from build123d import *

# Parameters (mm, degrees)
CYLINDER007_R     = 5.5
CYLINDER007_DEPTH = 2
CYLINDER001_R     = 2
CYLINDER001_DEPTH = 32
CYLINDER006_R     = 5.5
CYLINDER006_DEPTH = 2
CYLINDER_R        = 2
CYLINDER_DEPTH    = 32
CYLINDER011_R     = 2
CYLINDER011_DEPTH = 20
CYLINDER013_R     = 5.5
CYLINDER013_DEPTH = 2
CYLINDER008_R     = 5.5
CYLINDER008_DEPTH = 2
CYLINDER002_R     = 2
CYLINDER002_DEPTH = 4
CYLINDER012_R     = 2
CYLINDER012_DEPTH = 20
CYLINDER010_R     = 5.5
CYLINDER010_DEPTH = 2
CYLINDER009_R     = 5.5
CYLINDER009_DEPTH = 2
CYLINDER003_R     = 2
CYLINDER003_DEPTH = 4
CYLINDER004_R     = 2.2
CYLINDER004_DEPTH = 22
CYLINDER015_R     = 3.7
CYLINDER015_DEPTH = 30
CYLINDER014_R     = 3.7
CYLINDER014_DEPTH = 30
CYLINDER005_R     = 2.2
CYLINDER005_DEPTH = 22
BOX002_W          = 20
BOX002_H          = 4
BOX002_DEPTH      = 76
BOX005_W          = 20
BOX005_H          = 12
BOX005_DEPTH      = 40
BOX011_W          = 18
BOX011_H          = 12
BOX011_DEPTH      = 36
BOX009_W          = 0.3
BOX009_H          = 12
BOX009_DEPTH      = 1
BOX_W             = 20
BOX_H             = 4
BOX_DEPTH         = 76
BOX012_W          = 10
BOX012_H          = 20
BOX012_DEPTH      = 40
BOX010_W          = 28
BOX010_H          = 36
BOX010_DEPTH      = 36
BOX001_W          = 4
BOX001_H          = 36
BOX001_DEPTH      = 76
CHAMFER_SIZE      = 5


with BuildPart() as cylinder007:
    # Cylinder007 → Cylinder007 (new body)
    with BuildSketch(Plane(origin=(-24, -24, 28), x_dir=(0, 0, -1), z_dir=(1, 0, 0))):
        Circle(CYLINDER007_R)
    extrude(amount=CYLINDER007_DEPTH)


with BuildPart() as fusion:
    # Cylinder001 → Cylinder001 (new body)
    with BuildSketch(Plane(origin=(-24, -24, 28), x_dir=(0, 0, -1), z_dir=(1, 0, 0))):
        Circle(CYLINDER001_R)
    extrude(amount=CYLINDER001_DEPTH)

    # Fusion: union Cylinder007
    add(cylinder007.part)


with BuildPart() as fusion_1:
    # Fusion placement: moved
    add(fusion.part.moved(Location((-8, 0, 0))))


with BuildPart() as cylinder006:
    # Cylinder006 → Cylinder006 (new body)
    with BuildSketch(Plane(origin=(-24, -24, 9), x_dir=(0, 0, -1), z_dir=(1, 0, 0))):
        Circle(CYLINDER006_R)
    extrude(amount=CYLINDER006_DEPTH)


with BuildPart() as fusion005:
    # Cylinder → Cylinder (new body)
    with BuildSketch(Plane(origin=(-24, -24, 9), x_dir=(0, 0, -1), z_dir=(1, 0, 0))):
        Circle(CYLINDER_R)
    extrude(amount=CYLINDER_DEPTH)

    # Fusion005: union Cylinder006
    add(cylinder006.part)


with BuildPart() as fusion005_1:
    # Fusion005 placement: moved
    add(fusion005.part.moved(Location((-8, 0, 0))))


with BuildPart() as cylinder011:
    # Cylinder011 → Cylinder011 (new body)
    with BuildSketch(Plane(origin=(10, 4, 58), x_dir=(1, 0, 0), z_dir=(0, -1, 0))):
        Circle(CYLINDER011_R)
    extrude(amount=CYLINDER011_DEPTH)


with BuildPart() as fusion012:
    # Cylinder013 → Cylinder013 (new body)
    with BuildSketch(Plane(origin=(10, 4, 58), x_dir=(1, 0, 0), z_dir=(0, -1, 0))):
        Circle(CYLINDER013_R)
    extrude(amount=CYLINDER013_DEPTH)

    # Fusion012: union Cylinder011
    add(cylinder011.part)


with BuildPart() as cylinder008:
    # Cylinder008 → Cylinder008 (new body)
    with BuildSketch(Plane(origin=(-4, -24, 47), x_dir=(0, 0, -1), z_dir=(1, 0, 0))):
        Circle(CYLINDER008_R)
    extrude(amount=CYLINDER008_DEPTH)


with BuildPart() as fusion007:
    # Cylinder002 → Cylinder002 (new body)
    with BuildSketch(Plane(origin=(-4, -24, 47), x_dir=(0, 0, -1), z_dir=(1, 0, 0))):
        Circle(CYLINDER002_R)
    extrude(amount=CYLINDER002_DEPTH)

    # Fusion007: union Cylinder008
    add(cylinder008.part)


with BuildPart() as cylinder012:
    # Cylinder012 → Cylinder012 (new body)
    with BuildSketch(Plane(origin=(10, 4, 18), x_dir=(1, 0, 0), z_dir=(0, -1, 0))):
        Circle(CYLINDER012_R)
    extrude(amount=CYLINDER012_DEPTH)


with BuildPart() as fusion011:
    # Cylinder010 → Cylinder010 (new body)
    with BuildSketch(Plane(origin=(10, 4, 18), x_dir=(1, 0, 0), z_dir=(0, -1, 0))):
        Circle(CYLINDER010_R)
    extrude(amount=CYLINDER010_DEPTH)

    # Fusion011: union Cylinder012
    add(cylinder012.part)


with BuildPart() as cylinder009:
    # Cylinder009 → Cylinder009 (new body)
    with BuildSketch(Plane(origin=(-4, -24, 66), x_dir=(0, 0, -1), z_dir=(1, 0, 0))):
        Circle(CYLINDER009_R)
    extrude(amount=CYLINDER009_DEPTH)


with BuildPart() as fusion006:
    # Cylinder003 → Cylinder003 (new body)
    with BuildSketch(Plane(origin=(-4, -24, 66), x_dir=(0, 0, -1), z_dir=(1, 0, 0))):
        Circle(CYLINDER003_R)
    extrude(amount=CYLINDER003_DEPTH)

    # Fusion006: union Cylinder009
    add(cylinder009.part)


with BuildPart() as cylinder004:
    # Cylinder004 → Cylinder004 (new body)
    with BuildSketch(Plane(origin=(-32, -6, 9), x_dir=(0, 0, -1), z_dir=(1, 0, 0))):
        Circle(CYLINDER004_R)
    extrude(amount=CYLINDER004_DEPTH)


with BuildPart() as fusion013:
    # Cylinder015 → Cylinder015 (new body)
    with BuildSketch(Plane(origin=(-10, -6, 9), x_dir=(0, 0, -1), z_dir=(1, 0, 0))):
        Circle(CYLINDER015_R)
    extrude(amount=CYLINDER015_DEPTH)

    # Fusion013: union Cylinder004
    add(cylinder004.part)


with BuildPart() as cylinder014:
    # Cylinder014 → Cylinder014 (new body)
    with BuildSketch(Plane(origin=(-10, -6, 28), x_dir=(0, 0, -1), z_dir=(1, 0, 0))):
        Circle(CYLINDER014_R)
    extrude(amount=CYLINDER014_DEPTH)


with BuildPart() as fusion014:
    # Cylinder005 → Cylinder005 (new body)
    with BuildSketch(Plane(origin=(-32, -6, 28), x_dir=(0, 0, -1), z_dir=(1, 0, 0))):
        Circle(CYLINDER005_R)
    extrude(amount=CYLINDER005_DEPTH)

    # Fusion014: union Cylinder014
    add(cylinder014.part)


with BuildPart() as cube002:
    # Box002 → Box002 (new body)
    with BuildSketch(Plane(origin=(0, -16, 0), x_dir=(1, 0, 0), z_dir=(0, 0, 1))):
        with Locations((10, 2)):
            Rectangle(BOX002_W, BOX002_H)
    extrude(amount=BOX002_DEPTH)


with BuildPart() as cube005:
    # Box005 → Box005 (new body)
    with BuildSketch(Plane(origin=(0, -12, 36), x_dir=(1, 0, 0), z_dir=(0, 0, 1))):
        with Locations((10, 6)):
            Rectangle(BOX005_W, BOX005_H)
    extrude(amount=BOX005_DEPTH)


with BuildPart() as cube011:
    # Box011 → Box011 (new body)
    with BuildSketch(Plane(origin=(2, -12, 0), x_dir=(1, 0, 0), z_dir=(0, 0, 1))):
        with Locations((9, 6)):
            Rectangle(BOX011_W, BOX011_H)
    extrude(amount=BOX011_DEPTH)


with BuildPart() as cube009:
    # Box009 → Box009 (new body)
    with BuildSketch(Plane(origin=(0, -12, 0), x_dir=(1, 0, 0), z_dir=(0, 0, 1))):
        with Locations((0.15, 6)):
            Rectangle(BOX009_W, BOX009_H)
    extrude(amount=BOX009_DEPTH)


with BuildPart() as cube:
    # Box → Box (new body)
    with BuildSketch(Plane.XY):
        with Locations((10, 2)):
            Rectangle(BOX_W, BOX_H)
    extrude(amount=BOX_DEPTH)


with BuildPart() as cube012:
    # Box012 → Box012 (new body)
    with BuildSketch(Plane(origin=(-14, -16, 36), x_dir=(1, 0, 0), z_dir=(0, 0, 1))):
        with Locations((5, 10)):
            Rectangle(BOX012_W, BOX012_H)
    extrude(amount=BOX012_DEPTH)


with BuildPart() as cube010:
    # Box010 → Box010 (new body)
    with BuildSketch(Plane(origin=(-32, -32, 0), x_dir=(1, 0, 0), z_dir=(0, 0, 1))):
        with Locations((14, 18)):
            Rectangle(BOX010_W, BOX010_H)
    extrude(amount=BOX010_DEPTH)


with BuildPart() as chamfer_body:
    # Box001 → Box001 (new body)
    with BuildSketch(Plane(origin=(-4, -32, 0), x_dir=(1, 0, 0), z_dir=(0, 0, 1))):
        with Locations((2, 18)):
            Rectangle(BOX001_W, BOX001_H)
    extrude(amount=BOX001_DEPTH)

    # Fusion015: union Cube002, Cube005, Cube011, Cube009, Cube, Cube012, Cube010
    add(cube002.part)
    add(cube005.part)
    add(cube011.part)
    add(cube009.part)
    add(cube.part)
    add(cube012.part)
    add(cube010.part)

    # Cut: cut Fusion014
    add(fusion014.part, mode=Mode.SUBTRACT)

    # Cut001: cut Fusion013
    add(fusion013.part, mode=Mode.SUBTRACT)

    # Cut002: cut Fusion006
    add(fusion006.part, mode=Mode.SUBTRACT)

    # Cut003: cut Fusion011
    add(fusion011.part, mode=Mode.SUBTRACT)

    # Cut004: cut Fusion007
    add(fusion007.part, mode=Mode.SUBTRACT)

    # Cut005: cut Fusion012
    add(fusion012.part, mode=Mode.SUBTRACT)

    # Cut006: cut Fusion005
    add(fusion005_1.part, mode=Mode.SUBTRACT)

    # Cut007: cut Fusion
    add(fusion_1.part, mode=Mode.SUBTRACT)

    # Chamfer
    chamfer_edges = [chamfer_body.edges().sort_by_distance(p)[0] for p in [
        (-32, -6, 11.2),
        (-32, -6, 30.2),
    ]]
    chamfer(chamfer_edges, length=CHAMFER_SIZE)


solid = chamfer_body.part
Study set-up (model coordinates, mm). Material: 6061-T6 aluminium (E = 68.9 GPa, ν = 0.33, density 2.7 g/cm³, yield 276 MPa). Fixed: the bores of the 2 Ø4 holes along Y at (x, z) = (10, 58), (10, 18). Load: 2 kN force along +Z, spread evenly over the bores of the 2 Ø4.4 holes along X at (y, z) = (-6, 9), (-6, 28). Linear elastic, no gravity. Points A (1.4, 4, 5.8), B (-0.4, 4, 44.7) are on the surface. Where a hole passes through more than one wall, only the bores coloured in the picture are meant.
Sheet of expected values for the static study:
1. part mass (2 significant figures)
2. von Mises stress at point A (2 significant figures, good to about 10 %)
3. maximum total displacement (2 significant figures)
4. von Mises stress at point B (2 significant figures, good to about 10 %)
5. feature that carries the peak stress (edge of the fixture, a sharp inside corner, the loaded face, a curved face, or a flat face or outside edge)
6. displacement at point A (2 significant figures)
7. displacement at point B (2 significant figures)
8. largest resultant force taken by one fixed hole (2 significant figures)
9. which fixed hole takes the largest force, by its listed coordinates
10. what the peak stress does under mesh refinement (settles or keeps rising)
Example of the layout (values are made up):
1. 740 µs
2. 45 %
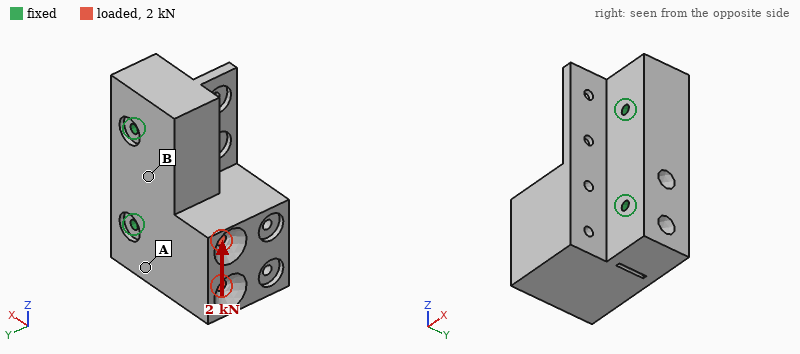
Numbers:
1. 210 g
2. 2.0 MPa
3. 9.6 µm
4. 5.6 MPa
5. edge of the fixture
6. 3.6 µm
7. 1.4 µm
8. 1.8 kN
9. (10, 58)
10. keeps rising
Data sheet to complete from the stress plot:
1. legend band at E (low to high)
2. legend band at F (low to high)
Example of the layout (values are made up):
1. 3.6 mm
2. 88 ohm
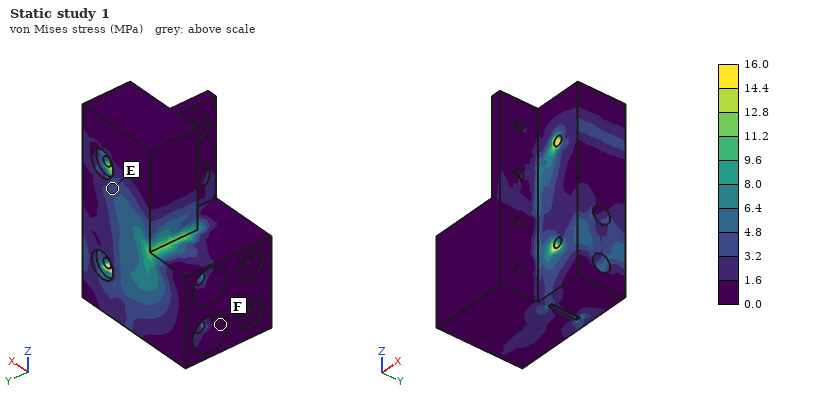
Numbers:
1. 3.2 to 4.8 MPa
2. 0.0 to 1.6 MPa
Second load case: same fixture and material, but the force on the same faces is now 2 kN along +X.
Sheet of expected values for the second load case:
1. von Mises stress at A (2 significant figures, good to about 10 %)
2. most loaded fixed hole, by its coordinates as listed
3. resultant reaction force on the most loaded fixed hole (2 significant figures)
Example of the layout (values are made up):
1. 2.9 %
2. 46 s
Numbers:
1. 3.0 MPa
2. (10, 18)
3. 1.9 kN
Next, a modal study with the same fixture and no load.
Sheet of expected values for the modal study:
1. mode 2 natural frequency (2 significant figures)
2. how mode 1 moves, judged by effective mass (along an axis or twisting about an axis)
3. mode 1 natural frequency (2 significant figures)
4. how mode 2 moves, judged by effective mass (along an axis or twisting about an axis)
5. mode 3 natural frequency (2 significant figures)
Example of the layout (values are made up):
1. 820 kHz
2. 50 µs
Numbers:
1. 8100 Hz
2. along Y
3. 4400 Hz
4. along Z
5. 11 kHz
